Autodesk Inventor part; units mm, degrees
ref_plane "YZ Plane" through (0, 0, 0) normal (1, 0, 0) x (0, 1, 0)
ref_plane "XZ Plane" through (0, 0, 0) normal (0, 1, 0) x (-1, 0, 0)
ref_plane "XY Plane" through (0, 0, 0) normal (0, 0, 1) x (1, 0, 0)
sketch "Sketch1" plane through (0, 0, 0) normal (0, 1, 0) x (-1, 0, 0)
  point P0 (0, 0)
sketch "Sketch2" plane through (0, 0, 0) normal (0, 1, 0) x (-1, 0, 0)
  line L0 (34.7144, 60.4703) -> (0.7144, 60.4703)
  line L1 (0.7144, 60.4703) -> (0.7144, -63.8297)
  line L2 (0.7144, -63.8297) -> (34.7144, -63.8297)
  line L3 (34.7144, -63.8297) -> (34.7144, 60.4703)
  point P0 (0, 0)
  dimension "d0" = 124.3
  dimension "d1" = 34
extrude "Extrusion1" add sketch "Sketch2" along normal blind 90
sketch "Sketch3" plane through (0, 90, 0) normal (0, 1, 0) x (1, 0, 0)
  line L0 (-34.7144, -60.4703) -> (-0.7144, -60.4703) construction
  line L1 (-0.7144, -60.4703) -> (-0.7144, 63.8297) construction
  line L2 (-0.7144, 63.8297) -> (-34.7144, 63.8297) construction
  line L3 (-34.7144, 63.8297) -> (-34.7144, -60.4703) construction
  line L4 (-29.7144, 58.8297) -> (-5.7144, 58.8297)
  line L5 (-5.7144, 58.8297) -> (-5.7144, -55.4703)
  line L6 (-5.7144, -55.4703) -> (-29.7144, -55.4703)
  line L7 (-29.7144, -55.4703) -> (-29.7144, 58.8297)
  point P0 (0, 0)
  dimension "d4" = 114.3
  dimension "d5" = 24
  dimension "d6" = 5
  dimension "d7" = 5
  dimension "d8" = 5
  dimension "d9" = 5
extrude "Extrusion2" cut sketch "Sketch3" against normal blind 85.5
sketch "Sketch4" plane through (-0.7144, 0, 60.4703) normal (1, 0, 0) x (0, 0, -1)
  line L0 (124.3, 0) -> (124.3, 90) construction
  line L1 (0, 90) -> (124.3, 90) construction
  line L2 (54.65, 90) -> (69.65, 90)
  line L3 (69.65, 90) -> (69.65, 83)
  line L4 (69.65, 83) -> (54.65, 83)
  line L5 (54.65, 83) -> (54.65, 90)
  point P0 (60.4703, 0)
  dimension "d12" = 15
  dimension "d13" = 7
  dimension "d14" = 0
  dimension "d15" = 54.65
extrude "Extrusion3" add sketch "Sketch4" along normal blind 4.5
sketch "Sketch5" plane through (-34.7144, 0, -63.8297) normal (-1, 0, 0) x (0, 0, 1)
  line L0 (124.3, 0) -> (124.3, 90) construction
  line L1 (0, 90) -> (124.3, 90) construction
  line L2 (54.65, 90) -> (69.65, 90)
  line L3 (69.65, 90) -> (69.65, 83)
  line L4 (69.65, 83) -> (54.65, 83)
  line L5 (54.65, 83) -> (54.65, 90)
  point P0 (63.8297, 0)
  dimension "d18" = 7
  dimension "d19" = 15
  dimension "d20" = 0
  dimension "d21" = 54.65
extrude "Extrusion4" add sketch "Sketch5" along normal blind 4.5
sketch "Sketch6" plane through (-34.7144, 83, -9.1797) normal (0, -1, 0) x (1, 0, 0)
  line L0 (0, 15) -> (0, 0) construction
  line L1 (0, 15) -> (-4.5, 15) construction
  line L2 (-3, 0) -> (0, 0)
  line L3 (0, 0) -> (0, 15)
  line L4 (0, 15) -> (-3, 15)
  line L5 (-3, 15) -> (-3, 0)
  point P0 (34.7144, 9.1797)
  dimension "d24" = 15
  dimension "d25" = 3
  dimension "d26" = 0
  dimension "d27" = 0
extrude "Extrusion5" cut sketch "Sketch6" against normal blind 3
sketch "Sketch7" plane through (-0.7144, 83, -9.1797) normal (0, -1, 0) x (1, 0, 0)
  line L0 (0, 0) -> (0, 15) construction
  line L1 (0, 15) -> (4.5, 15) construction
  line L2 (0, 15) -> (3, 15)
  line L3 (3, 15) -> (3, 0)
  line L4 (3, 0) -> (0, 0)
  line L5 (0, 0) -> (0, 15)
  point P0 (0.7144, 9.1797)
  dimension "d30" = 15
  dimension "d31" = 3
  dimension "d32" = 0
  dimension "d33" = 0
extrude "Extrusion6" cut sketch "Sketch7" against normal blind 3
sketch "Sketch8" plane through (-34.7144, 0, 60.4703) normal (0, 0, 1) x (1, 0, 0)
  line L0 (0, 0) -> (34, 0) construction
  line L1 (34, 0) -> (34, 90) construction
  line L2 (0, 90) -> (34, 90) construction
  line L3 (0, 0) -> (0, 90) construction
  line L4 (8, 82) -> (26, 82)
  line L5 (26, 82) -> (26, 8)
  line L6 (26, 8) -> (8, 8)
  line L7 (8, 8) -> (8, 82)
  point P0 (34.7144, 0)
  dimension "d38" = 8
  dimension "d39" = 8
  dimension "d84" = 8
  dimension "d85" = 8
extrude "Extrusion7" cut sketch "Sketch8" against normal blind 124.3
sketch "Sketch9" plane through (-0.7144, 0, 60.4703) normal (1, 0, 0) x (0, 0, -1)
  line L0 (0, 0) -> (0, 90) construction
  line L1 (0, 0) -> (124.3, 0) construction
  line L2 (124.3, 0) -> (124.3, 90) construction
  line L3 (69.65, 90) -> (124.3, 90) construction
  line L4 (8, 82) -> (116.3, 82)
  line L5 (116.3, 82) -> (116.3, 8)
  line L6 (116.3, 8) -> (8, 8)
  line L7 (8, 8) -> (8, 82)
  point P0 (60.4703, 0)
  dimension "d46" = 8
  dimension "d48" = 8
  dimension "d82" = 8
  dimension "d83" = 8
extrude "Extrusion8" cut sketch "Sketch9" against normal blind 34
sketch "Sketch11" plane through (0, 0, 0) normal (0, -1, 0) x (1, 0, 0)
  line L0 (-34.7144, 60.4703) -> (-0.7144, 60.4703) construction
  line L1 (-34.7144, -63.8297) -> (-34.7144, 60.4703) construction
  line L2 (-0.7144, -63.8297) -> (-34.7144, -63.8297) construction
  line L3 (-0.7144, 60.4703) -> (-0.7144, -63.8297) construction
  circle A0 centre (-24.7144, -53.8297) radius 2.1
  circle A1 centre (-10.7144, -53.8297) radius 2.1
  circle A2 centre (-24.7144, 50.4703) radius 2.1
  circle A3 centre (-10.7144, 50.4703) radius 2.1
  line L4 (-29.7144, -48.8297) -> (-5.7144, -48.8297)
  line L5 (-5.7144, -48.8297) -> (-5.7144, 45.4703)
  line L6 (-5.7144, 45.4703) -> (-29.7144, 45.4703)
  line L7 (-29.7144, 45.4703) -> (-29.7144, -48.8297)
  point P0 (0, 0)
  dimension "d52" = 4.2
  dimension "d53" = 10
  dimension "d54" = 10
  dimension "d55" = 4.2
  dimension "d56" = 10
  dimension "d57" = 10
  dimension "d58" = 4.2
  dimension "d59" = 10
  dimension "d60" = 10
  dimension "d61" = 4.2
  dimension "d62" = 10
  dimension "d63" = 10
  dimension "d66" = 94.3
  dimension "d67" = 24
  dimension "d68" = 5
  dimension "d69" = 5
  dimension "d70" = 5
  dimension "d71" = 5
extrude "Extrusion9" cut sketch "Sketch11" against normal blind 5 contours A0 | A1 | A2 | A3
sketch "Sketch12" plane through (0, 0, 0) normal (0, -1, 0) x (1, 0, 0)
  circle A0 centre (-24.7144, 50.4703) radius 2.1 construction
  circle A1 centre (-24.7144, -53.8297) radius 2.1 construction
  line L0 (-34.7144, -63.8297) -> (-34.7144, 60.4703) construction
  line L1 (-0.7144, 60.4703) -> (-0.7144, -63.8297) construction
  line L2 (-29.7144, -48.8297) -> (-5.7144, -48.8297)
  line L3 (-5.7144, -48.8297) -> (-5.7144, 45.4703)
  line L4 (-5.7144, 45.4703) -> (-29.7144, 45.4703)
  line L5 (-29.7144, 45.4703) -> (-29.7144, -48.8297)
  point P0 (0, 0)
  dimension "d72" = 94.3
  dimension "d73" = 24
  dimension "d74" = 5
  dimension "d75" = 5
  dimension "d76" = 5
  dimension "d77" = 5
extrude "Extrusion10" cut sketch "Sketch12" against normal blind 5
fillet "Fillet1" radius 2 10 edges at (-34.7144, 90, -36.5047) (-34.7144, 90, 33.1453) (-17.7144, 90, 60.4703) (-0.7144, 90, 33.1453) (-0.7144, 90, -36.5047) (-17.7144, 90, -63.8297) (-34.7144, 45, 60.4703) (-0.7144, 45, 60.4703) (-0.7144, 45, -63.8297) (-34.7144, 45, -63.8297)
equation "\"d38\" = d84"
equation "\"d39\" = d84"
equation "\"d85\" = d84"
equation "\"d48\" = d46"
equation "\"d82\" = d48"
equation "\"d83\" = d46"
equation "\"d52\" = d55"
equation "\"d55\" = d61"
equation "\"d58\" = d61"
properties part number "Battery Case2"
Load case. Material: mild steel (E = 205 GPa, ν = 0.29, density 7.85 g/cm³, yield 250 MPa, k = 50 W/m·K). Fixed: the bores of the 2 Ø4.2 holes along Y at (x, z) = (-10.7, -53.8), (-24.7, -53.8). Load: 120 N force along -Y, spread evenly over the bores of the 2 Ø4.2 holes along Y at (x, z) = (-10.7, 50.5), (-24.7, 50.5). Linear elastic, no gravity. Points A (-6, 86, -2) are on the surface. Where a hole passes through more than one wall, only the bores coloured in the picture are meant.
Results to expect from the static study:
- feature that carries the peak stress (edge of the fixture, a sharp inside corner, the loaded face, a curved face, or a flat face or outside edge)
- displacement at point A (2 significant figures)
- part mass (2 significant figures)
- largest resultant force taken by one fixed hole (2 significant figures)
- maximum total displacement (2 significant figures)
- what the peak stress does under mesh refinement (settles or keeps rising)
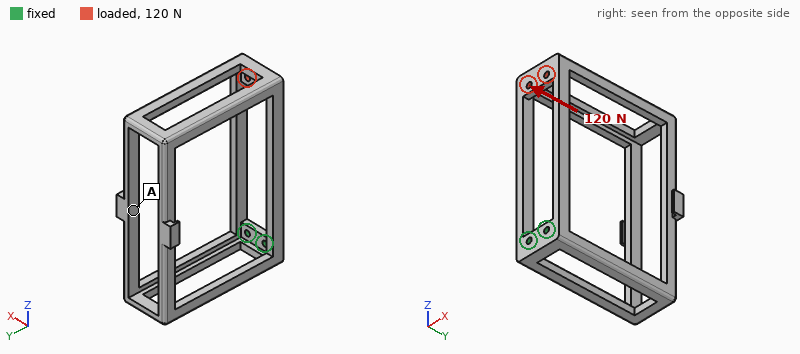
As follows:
edge of the fixture
0.25 mm
330 g
60 N
0.38 mm
keeps rising
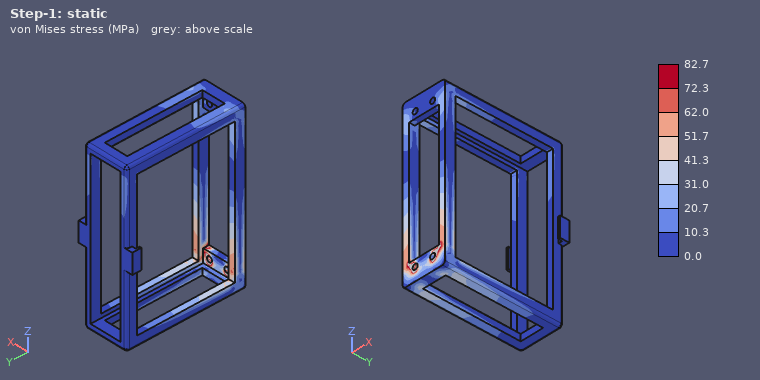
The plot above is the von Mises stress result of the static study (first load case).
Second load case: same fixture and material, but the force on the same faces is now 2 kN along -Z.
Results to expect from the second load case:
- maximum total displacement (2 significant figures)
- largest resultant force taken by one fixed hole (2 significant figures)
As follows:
92 µm
1.1 kN
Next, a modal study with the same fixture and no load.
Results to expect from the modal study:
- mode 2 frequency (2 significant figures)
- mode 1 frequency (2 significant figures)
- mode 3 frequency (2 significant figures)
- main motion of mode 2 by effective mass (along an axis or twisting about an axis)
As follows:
240 Hz
220 Hz
470 Hz
along X
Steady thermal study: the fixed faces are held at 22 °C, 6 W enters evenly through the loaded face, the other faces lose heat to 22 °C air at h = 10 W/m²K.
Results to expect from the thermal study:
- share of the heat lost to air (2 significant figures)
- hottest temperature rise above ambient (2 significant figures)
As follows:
73 %
55 K
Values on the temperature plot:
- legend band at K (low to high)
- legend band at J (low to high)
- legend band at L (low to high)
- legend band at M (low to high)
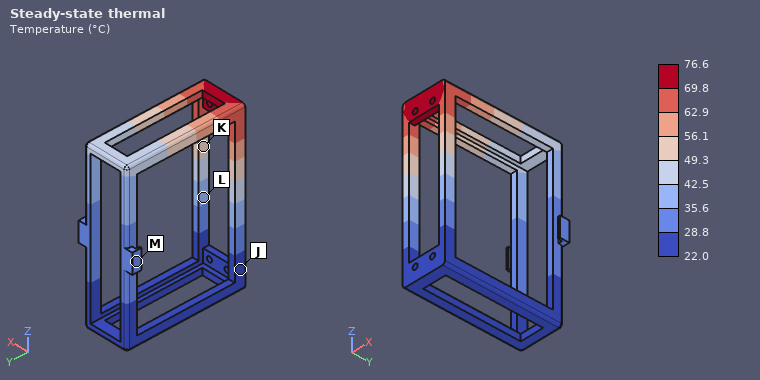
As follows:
49.3 to 56.1 °C
22.0 to 28.8 °C
35.6 to 42.5 °C
28.8 to 35.6 °C
